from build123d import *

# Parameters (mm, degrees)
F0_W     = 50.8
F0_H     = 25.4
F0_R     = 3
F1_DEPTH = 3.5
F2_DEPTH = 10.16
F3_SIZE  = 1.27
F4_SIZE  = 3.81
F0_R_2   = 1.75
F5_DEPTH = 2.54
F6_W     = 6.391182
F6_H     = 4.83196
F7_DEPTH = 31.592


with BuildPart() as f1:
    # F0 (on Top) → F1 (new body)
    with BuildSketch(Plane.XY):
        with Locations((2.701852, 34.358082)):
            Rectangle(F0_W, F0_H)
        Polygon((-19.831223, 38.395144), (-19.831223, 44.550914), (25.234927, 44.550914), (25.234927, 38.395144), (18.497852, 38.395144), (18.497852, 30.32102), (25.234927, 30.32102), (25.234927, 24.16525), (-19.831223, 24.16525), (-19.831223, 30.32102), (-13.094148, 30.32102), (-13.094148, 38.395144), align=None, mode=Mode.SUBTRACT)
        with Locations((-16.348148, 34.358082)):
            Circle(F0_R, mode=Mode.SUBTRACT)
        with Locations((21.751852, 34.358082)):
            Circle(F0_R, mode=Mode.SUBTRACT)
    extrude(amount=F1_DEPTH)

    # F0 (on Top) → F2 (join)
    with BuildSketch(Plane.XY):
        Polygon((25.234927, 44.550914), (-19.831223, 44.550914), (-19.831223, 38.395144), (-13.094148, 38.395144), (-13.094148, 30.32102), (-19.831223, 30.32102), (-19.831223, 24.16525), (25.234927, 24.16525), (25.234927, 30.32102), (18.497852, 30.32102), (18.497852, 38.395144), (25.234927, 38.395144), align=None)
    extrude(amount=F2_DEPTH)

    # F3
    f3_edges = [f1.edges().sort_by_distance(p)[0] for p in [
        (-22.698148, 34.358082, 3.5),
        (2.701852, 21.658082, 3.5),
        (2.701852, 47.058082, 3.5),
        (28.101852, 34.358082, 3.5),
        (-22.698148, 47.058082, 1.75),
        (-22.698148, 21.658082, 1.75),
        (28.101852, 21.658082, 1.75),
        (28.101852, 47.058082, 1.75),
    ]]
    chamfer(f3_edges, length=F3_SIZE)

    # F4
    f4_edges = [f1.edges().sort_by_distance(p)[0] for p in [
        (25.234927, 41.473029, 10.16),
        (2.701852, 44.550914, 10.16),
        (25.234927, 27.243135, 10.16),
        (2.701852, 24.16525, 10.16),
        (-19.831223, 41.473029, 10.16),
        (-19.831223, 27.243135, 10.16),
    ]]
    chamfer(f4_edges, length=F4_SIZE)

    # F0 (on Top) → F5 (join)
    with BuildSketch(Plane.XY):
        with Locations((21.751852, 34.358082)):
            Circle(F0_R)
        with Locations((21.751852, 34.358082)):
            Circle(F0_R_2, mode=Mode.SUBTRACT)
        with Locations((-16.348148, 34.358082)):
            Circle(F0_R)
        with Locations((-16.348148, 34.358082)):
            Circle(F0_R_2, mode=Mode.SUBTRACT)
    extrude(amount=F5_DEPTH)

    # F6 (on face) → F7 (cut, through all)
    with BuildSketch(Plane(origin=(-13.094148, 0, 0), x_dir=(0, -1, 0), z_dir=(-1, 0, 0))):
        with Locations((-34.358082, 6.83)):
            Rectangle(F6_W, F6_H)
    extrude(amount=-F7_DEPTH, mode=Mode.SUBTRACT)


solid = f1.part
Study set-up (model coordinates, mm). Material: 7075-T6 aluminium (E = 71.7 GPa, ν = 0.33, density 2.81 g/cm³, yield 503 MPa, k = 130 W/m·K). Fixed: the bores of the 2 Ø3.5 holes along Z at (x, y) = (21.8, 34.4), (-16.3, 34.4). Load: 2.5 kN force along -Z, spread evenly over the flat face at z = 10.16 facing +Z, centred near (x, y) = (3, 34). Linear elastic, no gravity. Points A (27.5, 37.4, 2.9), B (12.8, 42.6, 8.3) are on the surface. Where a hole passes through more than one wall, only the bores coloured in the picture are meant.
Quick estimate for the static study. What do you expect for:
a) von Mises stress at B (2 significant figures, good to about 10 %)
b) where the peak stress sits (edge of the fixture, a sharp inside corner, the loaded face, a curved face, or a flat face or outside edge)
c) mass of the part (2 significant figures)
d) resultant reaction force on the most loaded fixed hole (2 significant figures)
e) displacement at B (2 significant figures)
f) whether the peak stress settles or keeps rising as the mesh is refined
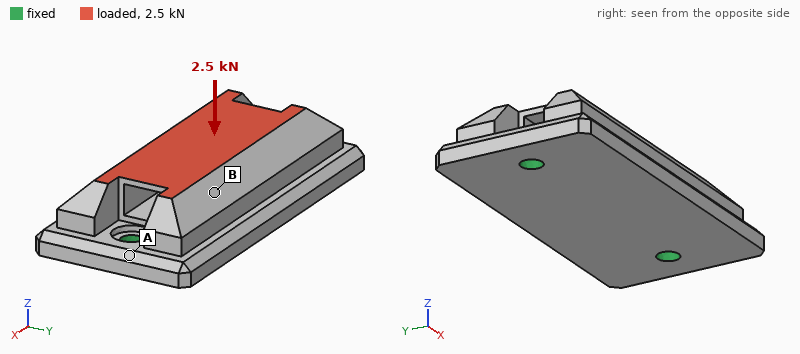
24 MPa
edge of the fixture
22 g
1.6 kN
17 µm
keeps rising
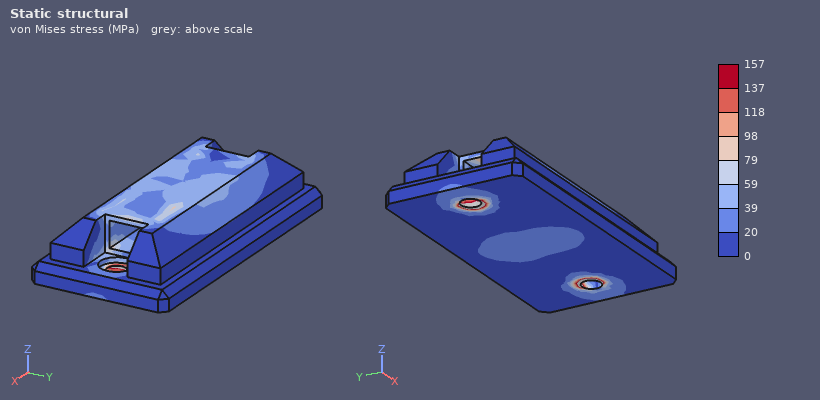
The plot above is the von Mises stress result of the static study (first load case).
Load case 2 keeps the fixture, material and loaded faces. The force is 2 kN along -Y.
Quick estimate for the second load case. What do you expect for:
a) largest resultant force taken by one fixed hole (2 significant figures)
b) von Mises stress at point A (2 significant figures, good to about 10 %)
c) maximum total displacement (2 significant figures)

1.0 kN
57 MPa
0.10 mm
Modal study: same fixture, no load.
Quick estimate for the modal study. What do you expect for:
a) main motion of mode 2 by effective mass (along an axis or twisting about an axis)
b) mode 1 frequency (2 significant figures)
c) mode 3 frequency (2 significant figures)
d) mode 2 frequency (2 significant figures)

along Z
6700 Hz
21 kHz
14 kHz
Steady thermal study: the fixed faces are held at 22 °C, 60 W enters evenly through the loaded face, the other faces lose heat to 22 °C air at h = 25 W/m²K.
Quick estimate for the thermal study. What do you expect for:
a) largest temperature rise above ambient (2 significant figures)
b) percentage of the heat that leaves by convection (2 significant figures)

44 K
3.7 %
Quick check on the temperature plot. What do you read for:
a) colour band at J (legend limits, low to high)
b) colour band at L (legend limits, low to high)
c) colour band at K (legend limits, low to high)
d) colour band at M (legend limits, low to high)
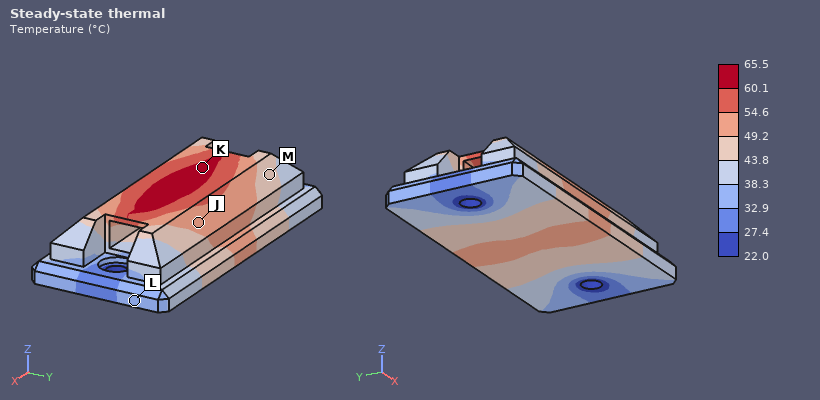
49.2 to 54.6 °C
32.9 to 38.3 °C
60.1 to 65.5 °C
43.8 to 49.2 °C
